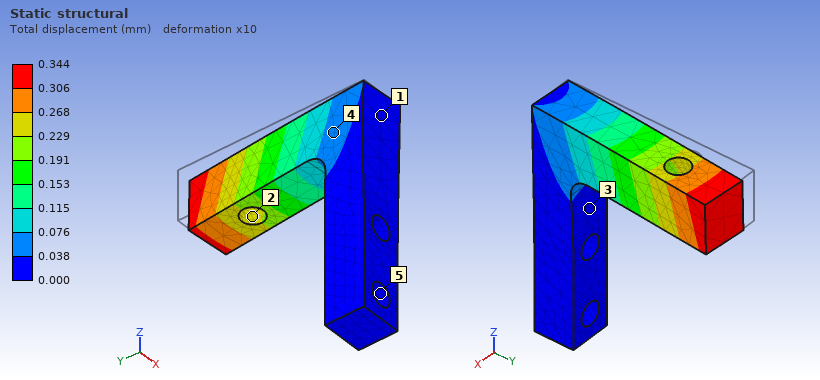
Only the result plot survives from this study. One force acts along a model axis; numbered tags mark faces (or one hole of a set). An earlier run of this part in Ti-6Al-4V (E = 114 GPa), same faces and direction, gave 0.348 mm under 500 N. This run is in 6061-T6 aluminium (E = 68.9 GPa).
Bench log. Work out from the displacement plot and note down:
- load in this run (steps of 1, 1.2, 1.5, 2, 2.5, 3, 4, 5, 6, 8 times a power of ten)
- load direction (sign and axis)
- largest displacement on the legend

300 N
+X
0.344 mm
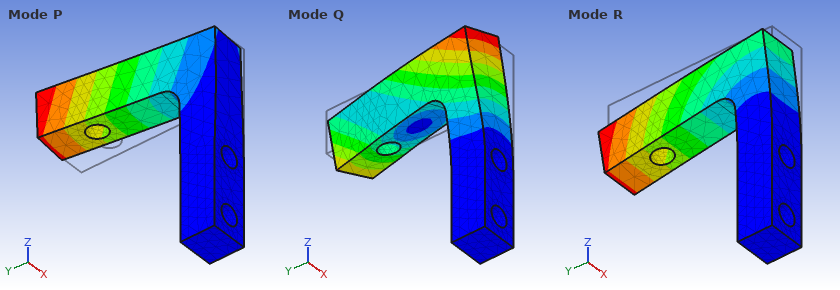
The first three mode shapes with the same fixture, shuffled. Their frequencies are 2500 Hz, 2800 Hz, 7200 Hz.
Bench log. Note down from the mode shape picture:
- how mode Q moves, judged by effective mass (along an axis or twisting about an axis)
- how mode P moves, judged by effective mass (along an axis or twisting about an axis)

along X
along X
